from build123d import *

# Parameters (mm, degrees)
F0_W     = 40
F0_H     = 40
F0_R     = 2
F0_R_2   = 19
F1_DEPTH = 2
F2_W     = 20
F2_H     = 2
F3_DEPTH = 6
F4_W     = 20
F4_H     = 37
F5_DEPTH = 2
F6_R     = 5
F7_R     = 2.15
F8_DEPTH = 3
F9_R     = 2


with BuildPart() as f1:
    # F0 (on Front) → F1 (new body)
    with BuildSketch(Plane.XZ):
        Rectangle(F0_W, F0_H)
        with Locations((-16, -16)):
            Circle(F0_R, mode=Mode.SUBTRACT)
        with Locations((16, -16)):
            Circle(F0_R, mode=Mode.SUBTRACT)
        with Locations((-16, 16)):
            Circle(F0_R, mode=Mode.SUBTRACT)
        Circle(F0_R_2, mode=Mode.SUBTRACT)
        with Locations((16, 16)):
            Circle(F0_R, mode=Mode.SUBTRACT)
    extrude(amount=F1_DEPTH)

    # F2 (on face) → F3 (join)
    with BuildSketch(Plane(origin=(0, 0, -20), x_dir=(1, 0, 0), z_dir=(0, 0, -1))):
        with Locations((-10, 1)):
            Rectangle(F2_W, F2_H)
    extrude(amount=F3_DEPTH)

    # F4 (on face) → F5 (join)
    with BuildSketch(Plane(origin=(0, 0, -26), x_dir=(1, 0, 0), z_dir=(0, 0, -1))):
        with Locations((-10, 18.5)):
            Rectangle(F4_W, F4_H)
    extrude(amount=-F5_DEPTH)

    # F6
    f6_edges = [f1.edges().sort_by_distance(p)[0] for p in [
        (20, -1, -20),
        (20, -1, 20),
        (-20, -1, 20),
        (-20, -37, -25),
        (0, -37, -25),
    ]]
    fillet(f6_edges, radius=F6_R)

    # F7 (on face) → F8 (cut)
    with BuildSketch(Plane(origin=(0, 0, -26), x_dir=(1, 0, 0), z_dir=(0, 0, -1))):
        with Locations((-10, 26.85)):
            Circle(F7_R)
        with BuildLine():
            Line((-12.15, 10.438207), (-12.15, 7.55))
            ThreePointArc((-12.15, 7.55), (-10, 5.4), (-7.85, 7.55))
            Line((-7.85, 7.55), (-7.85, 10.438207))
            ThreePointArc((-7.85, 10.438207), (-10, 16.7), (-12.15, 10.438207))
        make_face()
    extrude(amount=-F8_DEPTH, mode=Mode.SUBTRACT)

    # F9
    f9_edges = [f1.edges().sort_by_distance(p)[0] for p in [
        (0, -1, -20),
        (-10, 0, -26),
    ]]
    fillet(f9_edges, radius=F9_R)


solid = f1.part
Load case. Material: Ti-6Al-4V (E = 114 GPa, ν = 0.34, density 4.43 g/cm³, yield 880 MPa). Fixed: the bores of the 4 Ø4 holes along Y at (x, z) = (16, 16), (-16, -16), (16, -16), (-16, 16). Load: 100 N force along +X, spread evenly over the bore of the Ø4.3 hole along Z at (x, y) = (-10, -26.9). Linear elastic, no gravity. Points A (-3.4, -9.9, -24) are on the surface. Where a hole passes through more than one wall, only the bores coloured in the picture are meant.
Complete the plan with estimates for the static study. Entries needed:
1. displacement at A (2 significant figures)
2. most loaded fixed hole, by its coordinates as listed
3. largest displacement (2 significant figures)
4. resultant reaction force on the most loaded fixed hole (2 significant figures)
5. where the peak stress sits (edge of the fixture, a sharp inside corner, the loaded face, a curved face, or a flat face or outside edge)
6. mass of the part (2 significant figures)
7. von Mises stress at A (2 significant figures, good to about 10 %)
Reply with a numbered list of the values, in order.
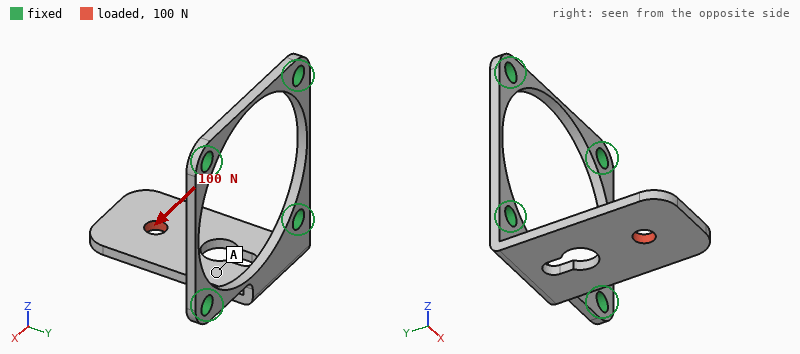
1. 0.12 mm
2. (-16, -16)
3. 0.33 mm
4. 86 N
5. a curved face
6. 10 g
7. 33 MPa
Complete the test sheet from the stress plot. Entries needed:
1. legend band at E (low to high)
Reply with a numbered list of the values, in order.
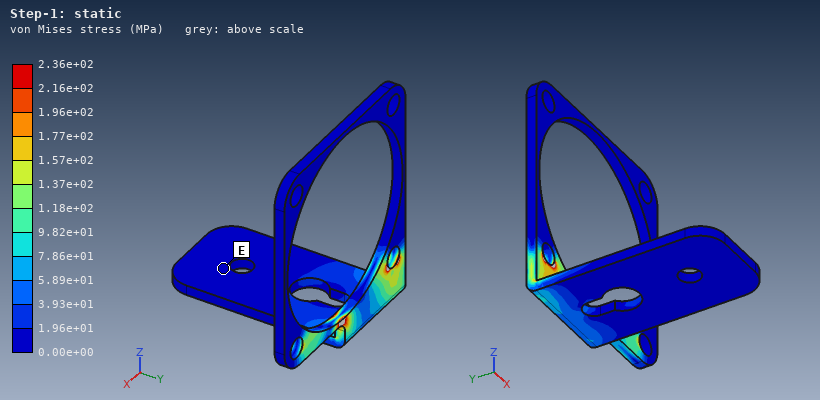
1. 0.00e+00 to 1.96e+01 MPa
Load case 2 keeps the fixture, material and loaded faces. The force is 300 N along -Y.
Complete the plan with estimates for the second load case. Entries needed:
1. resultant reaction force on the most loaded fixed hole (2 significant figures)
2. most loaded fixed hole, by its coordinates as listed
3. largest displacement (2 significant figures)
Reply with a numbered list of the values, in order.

1. 260 N
2. (-16, -16)
3. 0.46 mm
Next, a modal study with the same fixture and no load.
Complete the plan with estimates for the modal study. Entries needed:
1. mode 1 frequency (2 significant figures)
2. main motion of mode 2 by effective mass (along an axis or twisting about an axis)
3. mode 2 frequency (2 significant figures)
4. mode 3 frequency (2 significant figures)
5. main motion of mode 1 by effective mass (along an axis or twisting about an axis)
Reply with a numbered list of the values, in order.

1. 840 Hz
2. along X
3. 1700 Hz
4. 4200 Hz
5. along Z
